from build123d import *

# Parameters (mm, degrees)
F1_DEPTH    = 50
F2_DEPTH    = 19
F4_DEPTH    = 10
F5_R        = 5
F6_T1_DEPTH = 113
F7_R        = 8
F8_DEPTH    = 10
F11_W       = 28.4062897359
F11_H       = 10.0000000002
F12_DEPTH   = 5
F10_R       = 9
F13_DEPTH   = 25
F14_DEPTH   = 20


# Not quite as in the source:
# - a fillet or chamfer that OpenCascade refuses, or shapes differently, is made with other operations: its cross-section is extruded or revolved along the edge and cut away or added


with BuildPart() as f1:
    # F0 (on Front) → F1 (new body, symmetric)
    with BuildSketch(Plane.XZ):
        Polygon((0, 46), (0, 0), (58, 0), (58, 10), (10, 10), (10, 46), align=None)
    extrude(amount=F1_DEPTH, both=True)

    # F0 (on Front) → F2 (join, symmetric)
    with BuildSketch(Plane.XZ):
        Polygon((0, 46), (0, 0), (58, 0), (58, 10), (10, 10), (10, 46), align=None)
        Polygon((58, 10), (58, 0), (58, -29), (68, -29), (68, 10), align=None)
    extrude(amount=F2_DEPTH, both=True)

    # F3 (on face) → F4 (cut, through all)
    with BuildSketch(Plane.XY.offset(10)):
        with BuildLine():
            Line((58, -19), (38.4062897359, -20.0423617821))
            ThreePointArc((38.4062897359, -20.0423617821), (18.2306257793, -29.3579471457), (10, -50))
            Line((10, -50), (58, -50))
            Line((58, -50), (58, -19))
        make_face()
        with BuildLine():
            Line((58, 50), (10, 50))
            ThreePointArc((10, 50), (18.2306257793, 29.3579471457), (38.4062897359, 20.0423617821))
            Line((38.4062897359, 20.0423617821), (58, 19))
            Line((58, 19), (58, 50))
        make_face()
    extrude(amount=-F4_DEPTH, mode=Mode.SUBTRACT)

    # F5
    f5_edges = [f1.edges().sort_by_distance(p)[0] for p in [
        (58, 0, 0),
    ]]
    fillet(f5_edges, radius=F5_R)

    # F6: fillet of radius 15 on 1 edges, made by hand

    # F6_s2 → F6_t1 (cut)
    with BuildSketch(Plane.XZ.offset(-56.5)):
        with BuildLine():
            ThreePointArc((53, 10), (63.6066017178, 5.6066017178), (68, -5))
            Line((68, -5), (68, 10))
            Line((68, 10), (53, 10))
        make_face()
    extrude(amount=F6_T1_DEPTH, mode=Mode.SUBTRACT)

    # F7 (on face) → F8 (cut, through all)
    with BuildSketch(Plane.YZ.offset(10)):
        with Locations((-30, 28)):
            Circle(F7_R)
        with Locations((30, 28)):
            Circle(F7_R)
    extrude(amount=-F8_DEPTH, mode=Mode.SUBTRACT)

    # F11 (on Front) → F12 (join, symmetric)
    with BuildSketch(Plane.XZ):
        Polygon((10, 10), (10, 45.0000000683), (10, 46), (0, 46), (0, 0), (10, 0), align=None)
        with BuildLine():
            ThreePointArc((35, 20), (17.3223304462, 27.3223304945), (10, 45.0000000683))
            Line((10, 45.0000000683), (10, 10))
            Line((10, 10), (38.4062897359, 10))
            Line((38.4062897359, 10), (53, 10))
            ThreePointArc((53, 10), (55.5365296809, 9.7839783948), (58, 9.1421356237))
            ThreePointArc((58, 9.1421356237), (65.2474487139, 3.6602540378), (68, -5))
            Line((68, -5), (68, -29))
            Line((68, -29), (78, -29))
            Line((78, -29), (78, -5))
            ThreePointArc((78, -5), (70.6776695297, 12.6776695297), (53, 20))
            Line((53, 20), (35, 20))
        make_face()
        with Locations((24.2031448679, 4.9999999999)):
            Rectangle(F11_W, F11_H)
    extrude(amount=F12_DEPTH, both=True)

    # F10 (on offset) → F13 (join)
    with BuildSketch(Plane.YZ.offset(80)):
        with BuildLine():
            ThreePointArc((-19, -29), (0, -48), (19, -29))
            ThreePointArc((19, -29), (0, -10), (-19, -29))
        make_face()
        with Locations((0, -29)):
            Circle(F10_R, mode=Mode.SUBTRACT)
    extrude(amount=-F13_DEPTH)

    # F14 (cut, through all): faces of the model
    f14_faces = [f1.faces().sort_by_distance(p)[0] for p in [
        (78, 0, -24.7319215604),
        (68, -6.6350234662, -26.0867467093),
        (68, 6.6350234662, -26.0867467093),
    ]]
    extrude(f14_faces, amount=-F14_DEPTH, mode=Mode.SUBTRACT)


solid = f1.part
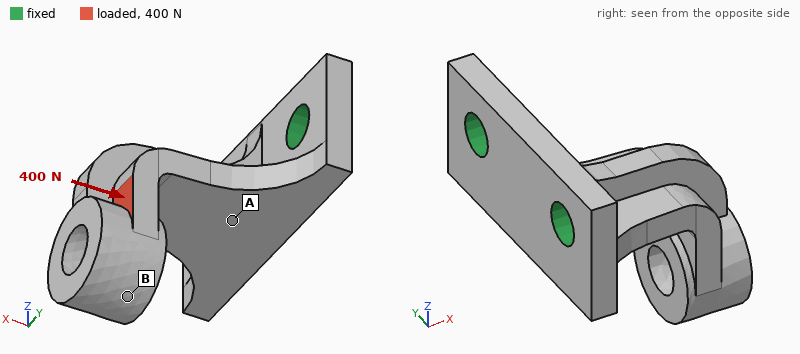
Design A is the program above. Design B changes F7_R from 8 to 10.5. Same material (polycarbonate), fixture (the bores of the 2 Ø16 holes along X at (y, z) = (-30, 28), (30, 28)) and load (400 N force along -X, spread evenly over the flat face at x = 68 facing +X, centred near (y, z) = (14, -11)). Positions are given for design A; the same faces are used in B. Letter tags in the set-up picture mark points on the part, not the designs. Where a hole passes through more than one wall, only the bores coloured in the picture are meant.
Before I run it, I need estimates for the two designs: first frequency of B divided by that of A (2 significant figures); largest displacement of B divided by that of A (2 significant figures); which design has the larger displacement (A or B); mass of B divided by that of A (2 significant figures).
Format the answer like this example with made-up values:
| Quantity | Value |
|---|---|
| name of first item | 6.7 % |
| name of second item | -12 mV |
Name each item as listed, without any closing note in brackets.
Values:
| Quantity | Value |
|---|---|
| first frequency of B divided by that of A | 1.1 |
| largest displacement of B divided by that of A | 0.89 |
| which design has the larger displacement | A |
| mass of B divided by that of A | 0.97 |
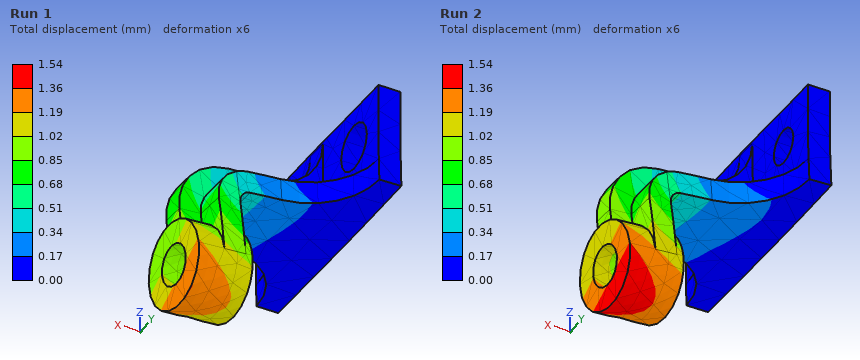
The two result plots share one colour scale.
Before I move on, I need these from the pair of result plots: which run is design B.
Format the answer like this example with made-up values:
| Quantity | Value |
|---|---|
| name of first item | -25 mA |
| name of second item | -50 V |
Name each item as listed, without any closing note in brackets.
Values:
| Quantity | Value |
|---|---|
| which run is design B | Run 1 |
